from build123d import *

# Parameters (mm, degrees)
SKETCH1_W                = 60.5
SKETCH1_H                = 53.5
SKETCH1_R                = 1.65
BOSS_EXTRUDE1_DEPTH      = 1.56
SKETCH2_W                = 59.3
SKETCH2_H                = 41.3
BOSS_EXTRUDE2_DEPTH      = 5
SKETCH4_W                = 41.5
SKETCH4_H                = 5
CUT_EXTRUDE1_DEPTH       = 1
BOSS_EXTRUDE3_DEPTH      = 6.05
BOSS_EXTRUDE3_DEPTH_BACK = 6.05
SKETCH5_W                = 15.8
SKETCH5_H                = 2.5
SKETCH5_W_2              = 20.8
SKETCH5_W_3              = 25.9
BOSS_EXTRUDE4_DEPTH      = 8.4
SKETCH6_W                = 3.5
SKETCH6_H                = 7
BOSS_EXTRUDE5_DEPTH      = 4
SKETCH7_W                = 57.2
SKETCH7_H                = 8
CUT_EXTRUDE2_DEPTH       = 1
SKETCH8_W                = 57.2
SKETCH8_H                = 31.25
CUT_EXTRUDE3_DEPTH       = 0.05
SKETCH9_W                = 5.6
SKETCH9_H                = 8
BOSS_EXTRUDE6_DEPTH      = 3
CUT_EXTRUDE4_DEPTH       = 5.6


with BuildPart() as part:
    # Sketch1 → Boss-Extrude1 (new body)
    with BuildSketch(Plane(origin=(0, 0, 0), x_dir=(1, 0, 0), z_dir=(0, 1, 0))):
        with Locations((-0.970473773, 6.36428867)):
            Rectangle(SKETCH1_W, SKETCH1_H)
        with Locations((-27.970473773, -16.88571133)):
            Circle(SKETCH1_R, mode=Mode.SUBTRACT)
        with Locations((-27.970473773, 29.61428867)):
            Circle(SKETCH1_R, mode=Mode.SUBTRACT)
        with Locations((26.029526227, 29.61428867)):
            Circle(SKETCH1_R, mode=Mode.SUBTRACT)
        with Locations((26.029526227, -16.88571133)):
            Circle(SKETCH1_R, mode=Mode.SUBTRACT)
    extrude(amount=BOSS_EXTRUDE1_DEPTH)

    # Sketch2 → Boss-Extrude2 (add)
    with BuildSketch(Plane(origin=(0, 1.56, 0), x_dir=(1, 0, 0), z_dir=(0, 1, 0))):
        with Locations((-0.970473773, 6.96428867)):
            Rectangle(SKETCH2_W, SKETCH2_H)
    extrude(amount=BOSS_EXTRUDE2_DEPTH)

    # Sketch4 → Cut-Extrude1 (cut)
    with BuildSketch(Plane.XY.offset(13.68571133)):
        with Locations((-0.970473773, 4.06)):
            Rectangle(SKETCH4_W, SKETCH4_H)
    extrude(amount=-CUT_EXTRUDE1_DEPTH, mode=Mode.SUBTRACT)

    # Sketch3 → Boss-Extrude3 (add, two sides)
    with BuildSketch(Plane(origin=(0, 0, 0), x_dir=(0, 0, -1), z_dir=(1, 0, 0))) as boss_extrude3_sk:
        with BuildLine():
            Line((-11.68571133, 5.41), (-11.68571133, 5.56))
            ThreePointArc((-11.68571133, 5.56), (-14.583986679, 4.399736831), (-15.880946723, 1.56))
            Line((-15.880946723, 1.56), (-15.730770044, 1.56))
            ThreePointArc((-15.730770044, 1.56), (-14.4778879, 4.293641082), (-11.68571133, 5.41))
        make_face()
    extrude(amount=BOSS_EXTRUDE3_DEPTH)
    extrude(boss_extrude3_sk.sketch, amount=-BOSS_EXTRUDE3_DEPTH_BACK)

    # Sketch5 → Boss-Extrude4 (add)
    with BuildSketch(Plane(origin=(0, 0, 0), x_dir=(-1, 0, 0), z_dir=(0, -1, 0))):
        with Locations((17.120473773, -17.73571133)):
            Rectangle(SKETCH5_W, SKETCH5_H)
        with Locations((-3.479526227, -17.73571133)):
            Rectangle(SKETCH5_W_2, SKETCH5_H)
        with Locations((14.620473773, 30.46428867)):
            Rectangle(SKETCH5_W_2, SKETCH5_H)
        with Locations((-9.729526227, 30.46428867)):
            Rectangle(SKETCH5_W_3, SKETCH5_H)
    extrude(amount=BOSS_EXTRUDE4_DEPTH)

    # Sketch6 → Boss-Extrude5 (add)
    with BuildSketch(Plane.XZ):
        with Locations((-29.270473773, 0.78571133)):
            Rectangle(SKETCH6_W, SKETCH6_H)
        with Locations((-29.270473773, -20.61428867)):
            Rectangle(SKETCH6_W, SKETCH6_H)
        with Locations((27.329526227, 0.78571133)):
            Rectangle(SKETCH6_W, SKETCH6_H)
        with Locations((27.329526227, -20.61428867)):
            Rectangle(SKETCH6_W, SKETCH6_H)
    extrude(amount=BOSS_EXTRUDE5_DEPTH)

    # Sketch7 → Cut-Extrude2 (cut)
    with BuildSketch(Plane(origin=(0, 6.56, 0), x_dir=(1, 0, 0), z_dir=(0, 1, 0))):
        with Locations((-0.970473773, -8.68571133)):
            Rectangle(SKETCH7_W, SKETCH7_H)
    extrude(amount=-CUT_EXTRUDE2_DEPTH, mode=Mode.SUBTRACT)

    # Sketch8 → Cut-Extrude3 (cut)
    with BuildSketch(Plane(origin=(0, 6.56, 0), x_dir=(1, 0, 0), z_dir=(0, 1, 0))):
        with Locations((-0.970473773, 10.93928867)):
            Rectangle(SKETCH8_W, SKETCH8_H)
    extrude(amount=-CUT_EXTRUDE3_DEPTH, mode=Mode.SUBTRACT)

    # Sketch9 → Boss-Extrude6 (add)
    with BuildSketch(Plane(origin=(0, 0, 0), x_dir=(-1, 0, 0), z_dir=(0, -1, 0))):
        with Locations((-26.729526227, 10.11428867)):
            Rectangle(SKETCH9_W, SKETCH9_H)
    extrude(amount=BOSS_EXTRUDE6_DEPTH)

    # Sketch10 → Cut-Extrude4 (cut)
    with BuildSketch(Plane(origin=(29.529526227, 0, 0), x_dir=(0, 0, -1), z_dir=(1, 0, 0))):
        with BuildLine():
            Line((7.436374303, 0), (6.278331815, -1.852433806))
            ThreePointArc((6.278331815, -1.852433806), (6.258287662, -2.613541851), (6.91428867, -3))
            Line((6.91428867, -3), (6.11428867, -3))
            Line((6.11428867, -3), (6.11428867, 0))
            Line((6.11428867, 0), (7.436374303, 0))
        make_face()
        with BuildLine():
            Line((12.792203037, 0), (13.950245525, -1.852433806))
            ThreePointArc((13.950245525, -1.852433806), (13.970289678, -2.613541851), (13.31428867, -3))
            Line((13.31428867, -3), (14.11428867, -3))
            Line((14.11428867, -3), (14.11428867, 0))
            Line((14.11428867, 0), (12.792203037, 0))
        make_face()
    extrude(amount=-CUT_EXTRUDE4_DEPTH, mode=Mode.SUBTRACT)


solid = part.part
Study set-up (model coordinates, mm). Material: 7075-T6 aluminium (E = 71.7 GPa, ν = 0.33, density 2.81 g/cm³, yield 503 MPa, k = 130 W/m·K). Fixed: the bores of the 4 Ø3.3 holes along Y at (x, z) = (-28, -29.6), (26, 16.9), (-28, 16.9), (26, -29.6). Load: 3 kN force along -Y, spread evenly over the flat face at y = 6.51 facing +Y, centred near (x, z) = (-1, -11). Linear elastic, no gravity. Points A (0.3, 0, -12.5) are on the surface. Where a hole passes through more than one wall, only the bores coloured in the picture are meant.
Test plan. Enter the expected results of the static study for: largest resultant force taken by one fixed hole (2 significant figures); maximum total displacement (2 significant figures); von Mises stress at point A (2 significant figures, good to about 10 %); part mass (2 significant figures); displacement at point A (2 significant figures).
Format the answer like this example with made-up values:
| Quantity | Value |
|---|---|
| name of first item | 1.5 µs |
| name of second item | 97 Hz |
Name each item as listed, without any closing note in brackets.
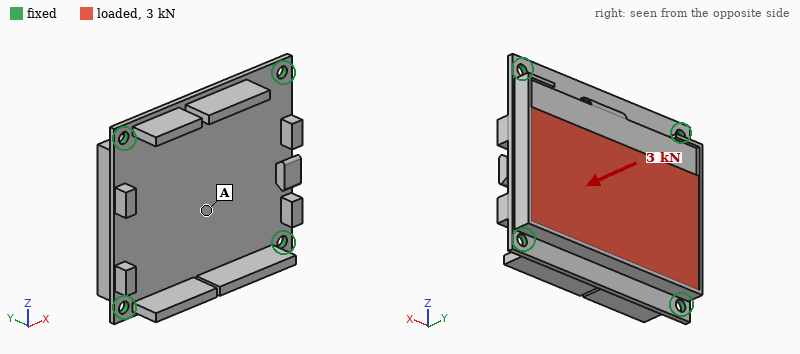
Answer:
| Quantity | Value |
|---|---|
| largest resultant force taken by one fixed hole | 1.5 kN |
| maximum total displacement | 83 µm |
| von Mises stress at point A | 34 MPa |
| part mass | 53 g |
| displacement at point A | 78 µm |
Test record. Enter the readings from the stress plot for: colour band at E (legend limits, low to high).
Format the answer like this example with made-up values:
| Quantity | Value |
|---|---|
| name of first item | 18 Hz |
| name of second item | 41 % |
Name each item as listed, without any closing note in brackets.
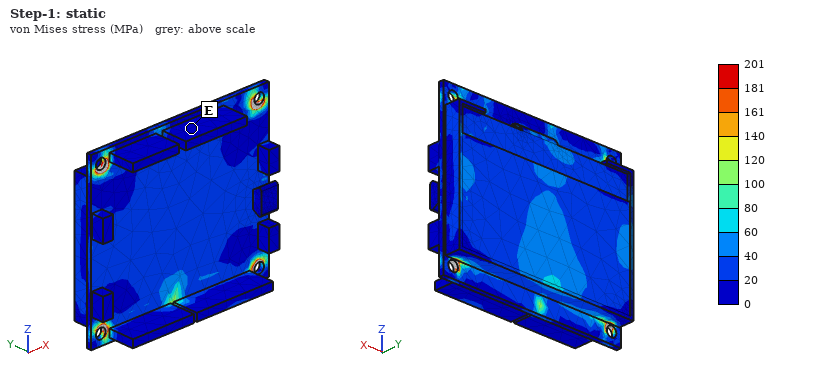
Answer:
| Quantity | Value |
|---|---|
| colour band at E | 0 to 20 MPa |
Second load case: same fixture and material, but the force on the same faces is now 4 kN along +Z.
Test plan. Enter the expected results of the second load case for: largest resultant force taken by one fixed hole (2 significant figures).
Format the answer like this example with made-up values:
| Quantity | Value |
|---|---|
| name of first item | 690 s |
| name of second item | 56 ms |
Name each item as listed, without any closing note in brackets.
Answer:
| Quantity | Value |
|---|---|
| largest resultant force taken by one fixed hole | 1.1 kN |
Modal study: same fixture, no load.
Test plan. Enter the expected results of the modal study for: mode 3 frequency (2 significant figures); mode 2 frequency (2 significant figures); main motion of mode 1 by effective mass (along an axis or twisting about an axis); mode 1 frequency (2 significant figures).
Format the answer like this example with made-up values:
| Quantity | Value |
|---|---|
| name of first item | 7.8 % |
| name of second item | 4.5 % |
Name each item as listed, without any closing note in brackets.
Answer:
| Quantity | Value |
|---|---|
| mode 3 frequency | 8300 Hz |
| mode 2 frequency | 6700 Hz |
| main motion of mode 1 by effective mass | along Y |
| mode 1 frequency | 4800 Hz |
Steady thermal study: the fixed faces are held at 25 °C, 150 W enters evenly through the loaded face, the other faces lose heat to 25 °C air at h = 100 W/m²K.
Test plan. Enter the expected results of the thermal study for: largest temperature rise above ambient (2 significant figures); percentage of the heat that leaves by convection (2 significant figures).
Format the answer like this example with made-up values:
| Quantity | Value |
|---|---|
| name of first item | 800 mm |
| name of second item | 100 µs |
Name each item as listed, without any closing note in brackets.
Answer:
| Quantity | Value |
|---|---|
| largest temperature rise above ambient | 74 K |
| percentage of the heat that leaves by convection | 28 % |
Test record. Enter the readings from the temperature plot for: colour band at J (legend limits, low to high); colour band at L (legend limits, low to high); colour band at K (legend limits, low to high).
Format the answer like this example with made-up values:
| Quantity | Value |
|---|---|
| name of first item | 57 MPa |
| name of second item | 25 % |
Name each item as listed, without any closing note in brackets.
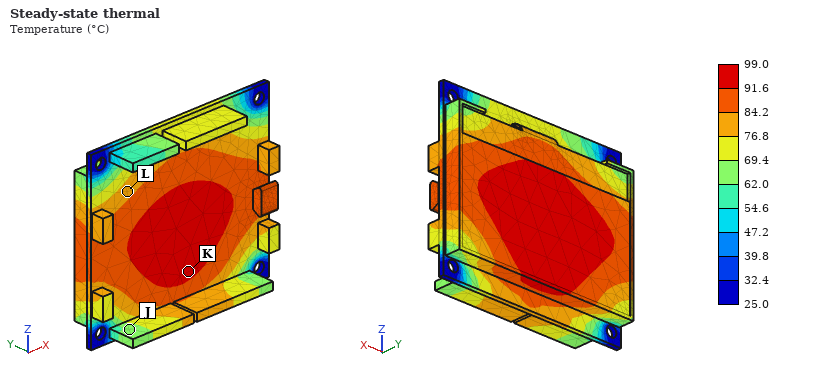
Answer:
| Quantity | Value |
|---|---|
| colour band at J | 62.0 to 69.4 °C |
| colour band at L | 76.8 to 84.2 °C |
| colour band at K | 91.6 to 99.0 °C |
